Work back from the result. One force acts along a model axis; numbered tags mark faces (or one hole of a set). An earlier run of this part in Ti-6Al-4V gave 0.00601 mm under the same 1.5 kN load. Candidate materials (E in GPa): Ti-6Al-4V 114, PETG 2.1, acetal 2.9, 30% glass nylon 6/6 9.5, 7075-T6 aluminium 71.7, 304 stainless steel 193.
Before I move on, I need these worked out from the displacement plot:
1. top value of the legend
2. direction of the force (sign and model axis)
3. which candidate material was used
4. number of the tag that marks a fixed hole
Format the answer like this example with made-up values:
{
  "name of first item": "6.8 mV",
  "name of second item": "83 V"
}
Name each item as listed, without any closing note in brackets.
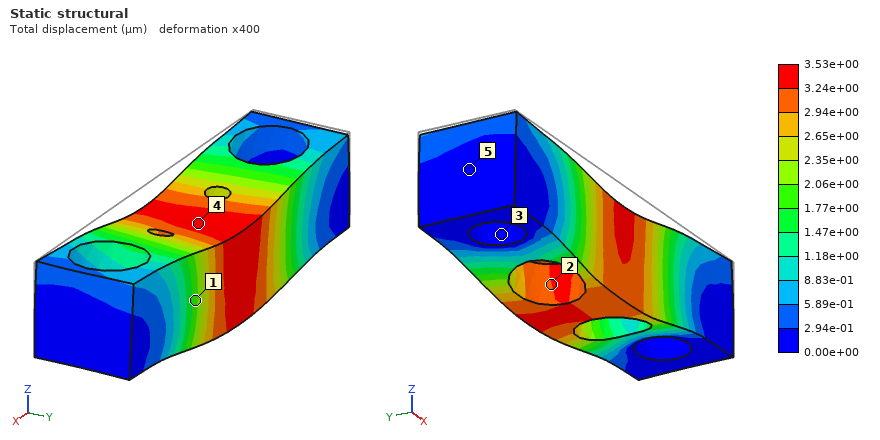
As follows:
{
  "top value of the legend": "3.53e+00 µm",
  "direction of the force": "-Z",
  "which candidate material was used": "304 stainless steel",
  "number of the tag that marks a fixed hole": "3"
}
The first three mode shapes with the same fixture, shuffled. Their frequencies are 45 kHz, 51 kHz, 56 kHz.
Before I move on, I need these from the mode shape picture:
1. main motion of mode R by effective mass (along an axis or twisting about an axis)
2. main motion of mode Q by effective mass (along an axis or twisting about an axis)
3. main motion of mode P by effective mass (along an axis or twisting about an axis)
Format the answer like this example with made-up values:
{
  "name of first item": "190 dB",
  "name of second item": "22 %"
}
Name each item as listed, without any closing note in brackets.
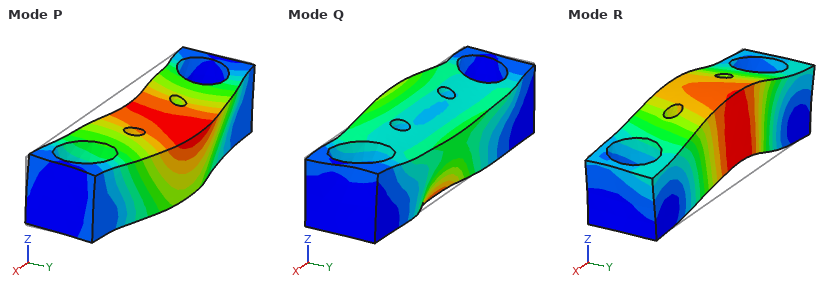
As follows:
{
  "main motion of mode R by effective mass": "along Z",
  "main motion of mode Q by effective mass": "twisting about X",
  "main motion of mode P by effective mass": "along Y"
}
